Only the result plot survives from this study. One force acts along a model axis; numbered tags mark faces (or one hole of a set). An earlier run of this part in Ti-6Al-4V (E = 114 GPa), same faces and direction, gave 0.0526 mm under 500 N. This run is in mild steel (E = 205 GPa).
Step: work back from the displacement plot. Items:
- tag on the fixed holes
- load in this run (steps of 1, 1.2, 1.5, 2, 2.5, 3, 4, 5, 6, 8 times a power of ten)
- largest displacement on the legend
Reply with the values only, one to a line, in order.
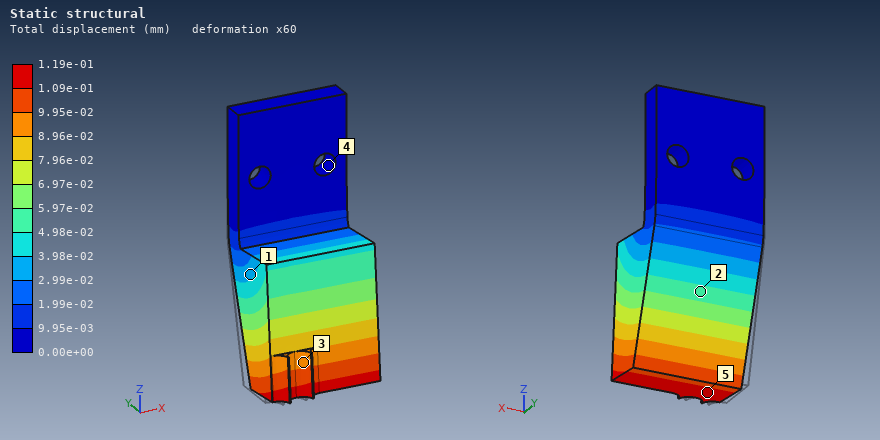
4
2 kN
1.19e-01 mm
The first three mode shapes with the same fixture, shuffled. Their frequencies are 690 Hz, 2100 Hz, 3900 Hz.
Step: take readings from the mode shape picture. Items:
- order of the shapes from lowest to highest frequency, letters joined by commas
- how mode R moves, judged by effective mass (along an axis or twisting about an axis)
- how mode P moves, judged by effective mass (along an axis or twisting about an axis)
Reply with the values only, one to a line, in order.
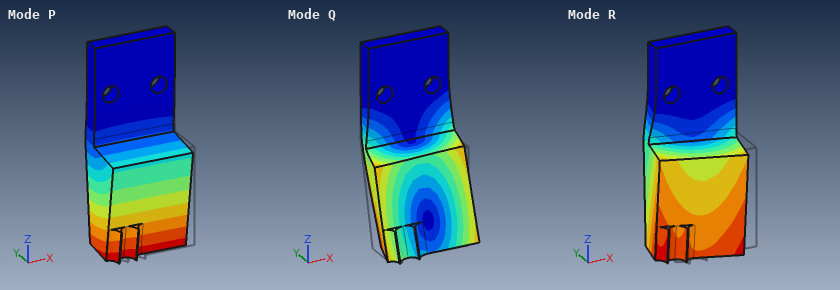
P, R, Q
along X
along Y
